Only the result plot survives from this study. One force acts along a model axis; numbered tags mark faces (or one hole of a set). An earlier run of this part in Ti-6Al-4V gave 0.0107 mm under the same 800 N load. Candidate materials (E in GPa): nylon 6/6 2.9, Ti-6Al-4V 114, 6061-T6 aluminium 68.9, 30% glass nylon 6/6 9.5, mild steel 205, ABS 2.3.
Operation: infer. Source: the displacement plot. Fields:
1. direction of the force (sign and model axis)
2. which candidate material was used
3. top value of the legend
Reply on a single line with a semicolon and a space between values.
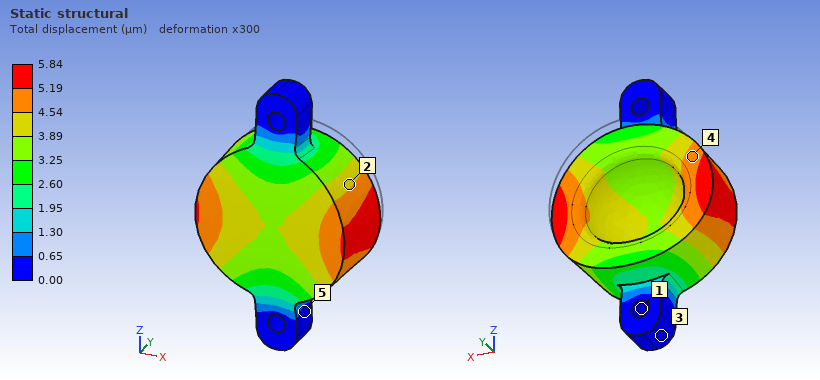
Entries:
-Y; mild steel; 5.84 µm
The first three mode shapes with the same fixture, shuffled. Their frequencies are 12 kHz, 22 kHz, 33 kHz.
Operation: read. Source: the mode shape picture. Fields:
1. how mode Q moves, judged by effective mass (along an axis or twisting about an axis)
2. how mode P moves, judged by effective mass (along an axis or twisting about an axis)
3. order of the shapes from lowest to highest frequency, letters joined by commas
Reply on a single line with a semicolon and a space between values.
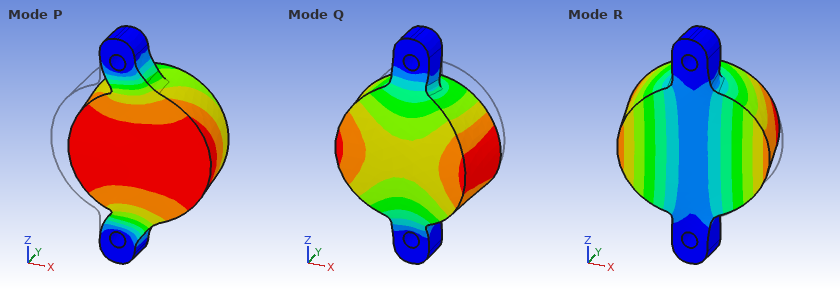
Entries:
along Y; along X; R, Q, P
